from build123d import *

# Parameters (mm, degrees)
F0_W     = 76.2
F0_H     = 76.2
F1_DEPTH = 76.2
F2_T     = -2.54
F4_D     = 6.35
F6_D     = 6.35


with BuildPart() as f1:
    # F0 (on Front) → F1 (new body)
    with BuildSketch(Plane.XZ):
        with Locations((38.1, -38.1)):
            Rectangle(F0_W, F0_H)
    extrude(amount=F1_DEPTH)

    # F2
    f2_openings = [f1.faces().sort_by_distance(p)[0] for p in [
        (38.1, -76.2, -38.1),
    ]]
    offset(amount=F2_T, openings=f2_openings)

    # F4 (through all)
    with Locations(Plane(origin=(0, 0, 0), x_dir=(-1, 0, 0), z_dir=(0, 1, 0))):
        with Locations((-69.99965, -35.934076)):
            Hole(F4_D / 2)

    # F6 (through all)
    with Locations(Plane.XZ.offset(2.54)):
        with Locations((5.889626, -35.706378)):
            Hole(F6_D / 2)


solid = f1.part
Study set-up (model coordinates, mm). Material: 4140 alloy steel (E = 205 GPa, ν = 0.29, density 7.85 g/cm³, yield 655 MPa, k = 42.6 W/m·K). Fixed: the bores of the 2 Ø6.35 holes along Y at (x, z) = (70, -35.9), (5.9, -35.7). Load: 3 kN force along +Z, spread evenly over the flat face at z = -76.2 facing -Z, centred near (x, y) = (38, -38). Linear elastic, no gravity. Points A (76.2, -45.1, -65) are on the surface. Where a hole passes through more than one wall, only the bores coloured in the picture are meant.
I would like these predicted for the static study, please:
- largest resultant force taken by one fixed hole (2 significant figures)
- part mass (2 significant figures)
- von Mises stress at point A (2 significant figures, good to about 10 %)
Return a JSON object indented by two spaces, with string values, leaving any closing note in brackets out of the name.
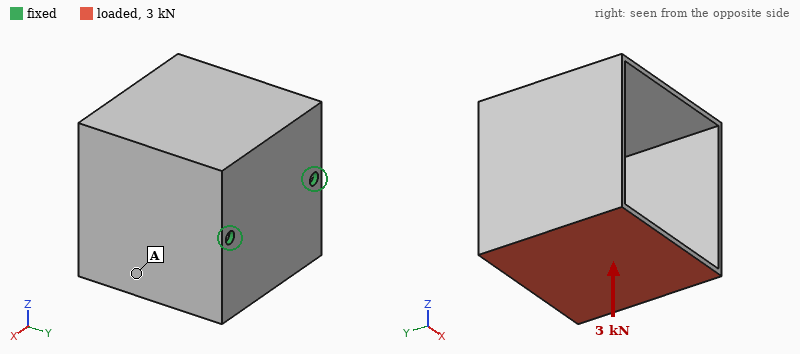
{
  "largest resultant force taken by one fixed hole": "1.5 kN",
  "part mass": "550 g",
  "von Mises stress at point A": "68 MPa"
}
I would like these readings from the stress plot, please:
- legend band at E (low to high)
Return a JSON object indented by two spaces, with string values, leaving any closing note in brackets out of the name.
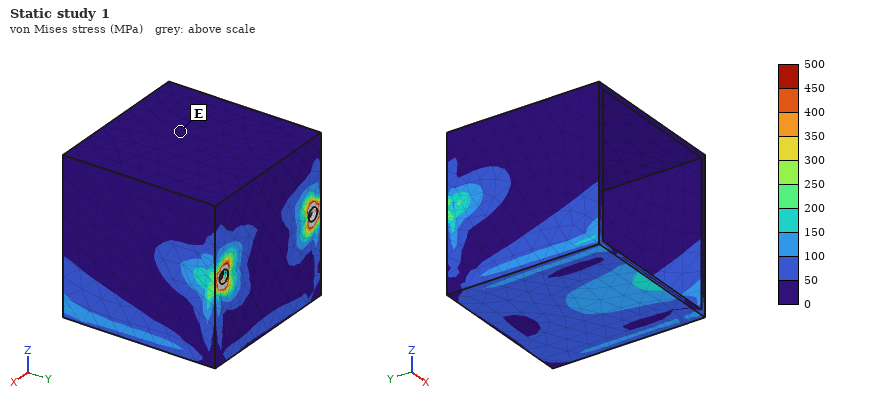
{
  "legend band at E": "0 to 50 MPa"
}
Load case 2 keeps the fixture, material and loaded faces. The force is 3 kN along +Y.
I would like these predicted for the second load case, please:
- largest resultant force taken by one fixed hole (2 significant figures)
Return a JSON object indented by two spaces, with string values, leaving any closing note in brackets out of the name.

{
  "largest resultant force taken by one fixed hole": "1.5 kN"
}
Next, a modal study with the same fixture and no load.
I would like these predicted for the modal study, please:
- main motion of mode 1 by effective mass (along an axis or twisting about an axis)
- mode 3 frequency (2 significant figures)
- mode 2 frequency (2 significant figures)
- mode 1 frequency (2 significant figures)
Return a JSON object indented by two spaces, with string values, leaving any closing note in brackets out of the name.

{
  "main motion of mode 1 by effective mass": "along Z",
  "mode 3 frequency": "1400 Hz",
  "mode 2 frequency": "850 Hz",
  "mode 1 frequency": "490 Hz"
}
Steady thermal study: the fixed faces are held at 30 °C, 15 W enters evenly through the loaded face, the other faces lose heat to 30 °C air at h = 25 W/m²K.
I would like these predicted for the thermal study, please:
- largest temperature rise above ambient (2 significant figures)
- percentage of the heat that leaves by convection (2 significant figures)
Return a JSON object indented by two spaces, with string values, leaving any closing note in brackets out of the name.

{
  "largest temperature rise above ambient": "31 K",
  "percentage of the heat that leaves by convection": "73 %"
}
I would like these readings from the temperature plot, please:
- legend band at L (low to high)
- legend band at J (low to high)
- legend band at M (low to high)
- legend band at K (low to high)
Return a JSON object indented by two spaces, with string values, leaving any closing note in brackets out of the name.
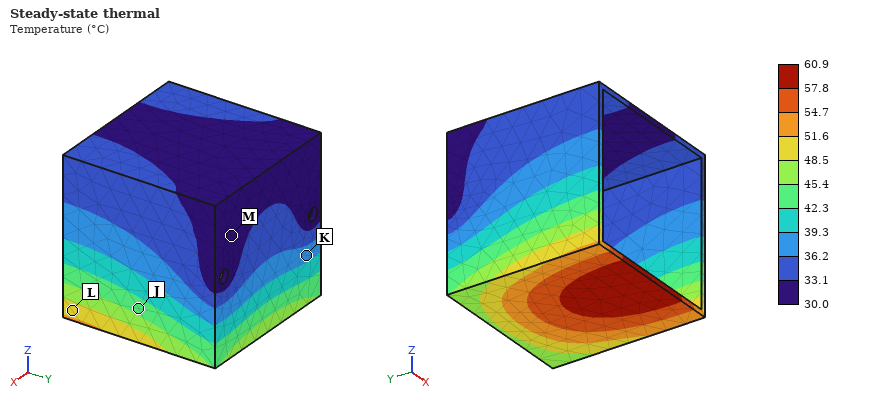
{
  "legend band at L": "48.5 to 51.6 °C",
  "legend band at J": "42.3 to 45.4 °C",
  "legend band at M": "30.0 to 33.1 °C",
  "legend band at K": "36.2 to 39.3 °C"
}
